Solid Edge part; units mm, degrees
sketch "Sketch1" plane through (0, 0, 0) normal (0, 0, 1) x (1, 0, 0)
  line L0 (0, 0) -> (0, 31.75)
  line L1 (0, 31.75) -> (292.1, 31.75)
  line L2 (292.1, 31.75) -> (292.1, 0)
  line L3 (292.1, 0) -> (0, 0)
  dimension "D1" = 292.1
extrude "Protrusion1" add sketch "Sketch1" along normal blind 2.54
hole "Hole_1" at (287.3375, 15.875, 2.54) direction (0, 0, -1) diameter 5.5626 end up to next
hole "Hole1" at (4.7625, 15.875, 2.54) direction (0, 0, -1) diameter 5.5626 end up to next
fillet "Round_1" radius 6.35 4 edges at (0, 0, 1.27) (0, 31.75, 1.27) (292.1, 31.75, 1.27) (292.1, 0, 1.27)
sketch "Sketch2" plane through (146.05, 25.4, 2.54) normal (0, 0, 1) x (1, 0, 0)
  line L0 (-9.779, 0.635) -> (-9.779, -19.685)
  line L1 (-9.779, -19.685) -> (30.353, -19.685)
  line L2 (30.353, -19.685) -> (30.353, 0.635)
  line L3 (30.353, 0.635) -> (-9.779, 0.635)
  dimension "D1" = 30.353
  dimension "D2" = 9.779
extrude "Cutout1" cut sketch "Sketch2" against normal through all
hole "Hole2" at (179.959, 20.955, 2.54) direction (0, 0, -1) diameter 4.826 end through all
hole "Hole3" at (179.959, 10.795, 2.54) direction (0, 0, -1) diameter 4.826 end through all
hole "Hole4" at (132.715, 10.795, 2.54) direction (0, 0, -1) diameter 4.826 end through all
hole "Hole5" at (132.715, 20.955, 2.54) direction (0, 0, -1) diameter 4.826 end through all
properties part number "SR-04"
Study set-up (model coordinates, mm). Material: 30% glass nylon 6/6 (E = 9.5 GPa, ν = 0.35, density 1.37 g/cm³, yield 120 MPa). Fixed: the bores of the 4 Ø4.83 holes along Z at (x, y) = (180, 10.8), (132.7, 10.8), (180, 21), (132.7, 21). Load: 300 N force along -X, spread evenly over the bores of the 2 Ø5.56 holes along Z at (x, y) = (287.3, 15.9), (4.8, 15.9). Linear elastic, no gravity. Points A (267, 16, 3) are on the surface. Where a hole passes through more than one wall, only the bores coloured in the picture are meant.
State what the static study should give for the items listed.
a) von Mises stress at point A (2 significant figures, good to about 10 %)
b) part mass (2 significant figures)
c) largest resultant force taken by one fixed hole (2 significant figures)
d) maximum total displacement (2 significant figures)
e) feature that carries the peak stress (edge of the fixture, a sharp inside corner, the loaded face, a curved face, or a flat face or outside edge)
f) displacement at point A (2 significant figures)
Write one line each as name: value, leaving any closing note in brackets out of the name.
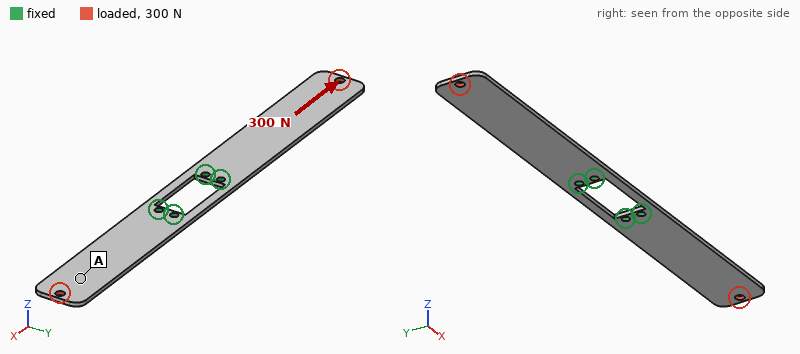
von Mises stress at point A: 2.2 MPa
part mass: 29 g
largest resultant force taken by one fixed hole: 75 N
maximum total displacement: 34 µm
feature that carries the peak stress: a flat face or outside edge
displacement at point A: 18 µm
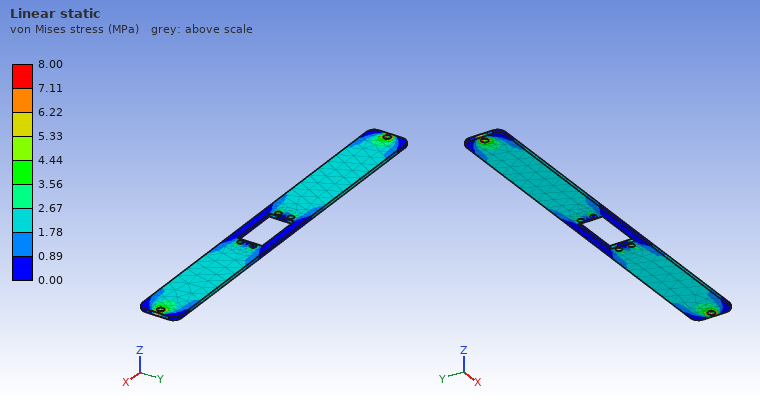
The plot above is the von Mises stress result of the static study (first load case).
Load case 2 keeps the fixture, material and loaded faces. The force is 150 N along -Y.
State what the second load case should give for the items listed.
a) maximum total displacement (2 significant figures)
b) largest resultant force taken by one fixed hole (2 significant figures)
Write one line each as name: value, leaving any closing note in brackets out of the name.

maximum total displacement: 1.1 mm
largest resultant force taken by one fixed hole: 440 N
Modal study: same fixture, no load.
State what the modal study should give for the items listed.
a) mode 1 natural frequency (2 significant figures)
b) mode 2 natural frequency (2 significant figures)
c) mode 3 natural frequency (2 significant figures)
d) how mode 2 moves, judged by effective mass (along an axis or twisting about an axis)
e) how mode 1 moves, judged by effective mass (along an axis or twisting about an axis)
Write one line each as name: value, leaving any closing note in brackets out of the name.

mode 1 natural frequency: 65 Hz
mode 2 natural frequency: 91 Hz
mode 3 natural frequency: 400 Hz
how mode 2 moves, judged by effective mass: along Z
how mode 1 moves, judged by effective mass: along Z
